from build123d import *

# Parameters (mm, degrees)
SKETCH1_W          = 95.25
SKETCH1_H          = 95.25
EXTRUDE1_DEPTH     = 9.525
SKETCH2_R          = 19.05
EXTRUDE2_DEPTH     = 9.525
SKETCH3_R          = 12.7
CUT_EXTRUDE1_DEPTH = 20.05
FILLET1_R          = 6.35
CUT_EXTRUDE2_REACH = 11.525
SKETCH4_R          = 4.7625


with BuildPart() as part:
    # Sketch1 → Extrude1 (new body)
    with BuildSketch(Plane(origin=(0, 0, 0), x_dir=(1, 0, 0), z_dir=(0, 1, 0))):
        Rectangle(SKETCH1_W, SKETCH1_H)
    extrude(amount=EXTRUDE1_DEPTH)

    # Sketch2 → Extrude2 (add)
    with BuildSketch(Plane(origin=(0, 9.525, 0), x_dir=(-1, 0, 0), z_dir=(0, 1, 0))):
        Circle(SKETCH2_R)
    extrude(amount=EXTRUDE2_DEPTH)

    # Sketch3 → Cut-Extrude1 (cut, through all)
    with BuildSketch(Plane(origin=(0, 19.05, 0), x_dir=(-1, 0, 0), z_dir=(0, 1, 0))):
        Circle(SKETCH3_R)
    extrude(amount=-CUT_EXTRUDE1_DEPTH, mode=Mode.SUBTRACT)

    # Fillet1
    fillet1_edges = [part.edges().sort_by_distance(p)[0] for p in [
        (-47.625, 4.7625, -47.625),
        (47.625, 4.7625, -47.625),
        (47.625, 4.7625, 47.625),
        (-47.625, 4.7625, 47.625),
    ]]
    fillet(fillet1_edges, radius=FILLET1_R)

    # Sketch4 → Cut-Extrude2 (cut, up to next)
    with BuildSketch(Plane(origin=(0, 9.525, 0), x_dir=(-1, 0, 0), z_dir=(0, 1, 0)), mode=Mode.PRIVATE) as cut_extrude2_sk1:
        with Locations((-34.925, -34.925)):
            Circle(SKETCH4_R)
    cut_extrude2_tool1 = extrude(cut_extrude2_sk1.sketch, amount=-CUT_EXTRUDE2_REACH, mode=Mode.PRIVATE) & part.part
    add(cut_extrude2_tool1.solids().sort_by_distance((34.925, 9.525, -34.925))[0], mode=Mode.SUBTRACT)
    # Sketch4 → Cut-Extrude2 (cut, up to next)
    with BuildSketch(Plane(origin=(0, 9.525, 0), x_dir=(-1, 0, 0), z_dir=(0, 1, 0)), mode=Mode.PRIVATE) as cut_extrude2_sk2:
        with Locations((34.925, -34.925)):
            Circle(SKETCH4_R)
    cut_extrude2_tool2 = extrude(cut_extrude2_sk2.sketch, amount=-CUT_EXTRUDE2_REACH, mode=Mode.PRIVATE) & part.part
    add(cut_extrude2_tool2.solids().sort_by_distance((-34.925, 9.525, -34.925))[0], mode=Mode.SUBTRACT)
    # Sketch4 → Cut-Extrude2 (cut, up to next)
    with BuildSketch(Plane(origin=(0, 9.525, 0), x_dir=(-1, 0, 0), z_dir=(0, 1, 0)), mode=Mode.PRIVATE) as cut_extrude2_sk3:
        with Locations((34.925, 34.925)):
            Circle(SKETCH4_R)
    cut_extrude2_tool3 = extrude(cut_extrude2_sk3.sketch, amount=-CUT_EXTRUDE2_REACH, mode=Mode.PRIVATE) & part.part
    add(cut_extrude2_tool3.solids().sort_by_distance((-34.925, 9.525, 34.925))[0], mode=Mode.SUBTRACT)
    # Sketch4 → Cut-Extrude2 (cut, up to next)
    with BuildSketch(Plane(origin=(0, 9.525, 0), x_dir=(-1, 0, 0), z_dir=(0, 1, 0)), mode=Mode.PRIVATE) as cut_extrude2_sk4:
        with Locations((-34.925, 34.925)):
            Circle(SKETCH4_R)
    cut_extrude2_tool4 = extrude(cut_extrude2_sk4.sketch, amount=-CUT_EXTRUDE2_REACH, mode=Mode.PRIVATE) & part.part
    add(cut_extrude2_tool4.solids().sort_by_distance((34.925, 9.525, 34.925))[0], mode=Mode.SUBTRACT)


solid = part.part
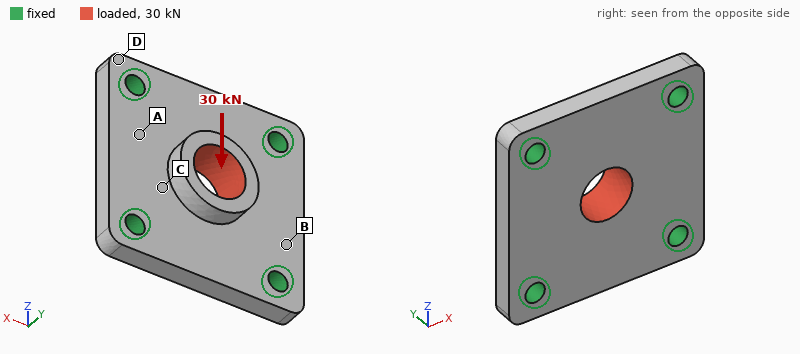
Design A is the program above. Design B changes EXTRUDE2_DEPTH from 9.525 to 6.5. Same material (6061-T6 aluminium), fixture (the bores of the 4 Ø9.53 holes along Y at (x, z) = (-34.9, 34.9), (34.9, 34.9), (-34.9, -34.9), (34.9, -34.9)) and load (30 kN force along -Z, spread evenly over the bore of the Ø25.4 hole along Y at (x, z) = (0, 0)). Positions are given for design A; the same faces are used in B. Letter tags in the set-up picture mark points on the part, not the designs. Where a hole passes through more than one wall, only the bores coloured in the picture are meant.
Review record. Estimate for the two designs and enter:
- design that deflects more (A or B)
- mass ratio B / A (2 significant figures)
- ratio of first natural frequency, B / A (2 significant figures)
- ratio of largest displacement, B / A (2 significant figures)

A
0.98
1.0
0.75
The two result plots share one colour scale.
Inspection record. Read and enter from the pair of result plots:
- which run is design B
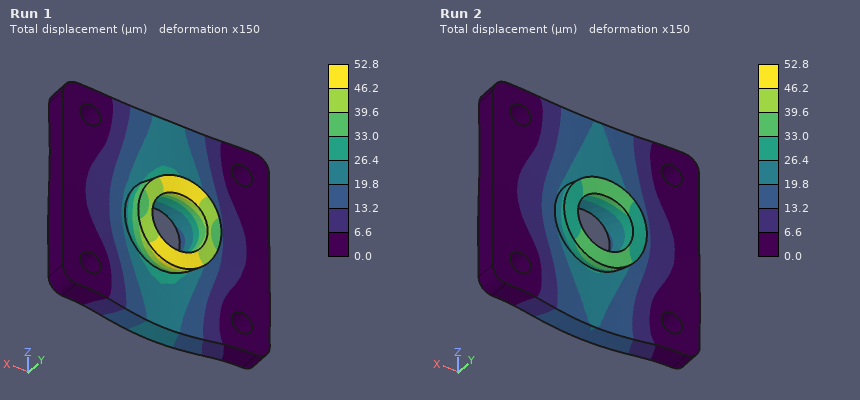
Run 2
